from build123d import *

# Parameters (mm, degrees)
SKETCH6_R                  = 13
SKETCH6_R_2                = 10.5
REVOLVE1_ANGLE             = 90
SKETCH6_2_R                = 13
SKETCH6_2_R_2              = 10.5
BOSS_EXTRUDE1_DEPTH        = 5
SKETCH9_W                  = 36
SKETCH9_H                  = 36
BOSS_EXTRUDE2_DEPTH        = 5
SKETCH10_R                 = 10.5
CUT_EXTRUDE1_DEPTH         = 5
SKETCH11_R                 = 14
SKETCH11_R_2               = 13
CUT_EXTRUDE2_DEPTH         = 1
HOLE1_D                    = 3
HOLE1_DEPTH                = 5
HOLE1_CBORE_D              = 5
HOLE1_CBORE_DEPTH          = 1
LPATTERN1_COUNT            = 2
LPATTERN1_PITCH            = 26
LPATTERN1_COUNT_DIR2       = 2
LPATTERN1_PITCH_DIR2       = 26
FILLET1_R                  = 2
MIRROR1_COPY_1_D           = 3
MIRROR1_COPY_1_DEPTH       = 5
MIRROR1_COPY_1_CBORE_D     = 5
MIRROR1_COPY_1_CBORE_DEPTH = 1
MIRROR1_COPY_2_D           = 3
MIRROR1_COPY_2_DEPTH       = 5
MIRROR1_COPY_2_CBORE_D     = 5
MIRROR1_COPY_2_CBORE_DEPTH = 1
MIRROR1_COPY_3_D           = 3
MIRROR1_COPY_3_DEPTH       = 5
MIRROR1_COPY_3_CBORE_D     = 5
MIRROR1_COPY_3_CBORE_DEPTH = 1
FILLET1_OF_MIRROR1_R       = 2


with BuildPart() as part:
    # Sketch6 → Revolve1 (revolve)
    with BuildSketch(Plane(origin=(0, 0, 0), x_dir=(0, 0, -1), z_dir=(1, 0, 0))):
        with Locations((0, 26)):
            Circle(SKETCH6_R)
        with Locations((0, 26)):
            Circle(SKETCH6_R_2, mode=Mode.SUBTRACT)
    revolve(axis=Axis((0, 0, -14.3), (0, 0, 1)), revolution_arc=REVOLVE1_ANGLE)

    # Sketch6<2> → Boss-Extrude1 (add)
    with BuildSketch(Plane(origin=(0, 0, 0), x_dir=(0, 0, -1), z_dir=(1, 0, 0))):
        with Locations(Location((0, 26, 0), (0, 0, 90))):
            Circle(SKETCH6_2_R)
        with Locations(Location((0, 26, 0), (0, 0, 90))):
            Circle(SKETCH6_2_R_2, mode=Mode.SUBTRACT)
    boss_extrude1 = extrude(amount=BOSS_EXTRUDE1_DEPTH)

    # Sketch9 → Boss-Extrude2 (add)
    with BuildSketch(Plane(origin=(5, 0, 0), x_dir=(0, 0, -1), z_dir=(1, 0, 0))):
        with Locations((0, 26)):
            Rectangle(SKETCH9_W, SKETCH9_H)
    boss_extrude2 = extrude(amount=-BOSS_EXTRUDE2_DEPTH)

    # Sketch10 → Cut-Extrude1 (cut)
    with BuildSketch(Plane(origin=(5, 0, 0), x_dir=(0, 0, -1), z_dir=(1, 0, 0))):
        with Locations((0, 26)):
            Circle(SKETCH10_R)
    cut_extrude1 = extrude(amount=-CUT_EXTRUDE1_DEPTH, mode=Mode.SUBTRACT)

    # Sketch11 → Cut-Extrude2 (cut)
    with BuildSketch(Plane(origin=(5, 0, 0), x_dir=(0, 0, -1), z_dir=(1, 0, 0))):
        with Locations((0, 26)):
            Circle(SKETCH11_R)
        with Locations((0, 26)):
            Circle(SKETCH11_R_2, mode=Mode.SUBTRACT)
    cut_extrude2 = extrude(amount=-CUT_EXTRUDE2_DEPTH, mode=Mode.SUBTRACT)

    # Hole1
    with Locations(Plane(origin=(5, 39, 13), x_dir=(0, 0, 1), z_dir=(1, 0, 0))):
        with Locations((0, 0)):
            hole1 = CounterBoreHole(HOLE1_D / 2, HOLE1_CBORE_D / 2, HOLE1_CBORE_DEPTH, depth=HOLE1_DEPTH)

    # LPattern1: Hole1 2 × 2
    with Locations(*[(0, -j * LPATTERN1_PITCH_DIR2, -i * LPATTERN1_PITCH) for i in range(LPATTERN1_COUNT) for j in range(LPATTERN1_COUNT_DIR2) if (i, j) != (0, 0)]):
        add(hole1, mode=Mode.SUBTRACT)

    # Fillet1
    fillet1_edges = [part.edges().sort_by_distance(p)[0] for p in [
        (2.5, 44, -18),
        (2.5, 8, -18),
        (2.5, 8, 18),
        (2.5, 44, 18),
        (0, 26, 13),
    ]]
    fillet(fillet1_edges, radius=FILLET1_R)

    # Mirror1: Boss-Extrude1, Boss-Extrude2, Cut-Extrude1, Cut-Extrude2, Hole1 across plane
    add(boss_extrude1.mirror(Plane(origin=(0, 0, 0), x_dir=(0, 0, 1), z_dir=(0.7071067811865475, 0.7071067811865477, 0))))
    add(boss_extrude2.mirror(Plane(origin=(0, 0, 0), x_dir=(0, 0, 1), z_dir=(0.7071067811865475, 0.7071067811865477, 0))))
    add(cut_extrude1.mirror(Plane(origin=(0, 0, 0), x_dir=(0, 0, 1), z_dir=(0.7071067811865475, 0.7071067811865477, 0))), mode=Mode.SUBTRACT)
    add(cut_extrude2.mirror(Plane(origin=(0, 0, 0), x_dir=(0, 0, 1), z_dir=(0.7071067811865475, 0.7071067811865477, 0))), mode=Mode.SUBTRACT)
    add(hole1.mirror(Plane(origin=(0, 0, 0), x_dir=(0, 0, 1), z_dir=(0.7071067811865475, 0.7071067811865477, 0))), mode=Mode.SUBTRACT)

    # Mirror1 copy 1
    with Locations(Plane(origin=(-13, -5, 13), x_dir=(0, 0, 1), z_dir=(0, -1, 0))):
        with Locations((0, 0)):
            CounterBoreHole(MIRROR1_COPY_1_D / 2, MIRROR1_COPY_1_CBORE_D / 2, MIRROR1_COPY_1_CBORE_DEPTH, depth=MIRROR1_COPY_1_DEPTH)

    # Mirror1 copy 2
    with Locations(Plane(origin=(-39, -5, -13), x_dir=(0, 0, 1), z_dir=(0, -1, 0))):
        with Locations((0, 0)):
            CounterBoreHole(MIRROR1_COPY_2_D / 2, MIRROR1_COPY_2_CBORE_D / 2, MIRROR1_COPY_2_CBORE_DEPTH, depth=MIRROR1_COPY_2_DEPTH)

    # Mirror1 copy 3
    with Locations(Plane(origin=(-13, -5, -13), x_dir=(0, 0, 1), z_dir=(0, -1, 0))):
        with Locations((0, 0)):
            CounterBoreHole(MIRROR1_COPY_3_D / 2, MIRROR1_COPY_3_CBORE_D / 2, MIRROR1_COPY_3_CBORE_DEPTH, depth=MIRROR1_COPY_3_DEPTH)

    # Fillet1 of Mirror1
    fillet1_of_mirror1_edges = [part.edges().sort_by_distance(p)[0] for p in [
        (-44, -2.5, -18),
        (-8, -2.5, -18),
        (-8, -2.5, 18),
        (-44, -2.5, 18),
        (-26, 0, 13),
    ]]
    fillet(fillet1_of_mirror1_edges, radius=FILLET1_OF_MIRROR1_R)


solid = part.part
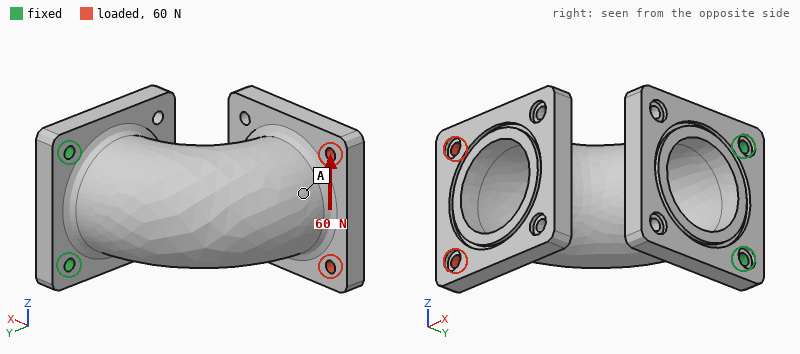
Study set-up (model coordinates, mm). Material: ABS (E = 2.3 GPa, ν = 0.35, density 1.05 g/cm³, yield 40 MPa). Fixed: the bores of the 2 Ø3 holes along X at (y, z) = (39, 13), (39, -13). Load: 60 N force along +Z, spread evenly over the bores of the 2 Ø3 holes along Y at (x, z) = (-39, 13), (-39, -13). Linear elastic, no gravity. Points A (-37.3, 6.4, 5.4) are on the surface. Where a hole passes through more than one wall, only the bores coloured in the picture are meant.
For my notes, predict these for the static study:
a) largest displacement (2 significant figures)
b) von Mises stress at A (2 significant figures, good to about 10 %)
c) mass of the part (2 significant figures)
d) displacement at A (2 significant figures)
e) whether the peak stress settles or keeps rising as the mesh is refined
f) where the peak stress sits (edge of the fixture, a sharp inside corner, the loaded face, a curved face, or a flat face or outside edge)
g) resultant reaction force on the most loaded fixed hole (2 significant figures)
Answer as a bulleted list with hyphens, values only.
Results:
- 0.41 mm
- 1.3 MPa
- 17 g
- 0.31 mm
- keeps rising
- edge of the fixture
- 140 N
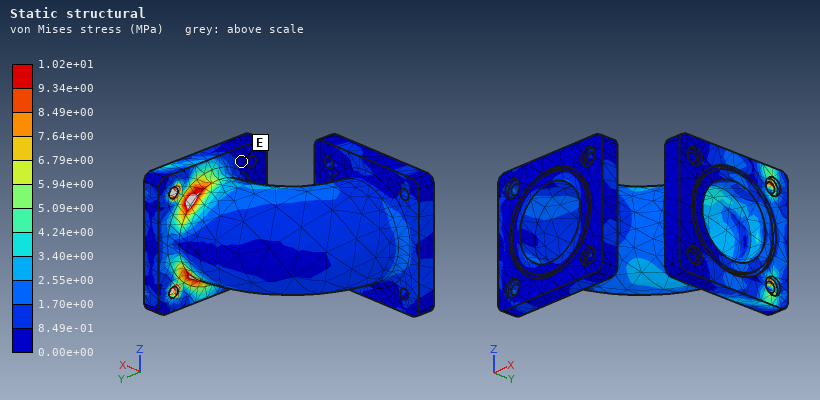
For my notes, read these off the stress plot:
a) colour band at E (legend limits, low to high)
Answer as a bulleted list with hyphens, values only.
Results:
- 0.00e+00 to 8.49e-01 MPa
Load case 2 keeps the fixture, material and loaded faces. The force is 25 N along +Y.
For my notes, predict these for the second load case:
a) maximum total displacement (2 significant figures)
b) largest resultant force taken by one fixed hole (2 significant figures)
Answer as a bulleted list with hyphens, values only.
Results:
- 0.94 mm
- 13 N
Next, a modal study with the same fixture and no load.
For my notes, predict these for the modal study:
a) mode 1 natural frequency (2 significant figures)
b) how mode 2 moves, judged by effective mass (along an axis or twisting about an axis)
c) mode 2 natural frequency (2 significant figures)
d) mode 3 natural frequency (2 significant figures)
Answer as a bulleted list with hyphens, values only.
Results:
- 300 Hz
- along Z
- 900 Hz
- 1800 Hz
